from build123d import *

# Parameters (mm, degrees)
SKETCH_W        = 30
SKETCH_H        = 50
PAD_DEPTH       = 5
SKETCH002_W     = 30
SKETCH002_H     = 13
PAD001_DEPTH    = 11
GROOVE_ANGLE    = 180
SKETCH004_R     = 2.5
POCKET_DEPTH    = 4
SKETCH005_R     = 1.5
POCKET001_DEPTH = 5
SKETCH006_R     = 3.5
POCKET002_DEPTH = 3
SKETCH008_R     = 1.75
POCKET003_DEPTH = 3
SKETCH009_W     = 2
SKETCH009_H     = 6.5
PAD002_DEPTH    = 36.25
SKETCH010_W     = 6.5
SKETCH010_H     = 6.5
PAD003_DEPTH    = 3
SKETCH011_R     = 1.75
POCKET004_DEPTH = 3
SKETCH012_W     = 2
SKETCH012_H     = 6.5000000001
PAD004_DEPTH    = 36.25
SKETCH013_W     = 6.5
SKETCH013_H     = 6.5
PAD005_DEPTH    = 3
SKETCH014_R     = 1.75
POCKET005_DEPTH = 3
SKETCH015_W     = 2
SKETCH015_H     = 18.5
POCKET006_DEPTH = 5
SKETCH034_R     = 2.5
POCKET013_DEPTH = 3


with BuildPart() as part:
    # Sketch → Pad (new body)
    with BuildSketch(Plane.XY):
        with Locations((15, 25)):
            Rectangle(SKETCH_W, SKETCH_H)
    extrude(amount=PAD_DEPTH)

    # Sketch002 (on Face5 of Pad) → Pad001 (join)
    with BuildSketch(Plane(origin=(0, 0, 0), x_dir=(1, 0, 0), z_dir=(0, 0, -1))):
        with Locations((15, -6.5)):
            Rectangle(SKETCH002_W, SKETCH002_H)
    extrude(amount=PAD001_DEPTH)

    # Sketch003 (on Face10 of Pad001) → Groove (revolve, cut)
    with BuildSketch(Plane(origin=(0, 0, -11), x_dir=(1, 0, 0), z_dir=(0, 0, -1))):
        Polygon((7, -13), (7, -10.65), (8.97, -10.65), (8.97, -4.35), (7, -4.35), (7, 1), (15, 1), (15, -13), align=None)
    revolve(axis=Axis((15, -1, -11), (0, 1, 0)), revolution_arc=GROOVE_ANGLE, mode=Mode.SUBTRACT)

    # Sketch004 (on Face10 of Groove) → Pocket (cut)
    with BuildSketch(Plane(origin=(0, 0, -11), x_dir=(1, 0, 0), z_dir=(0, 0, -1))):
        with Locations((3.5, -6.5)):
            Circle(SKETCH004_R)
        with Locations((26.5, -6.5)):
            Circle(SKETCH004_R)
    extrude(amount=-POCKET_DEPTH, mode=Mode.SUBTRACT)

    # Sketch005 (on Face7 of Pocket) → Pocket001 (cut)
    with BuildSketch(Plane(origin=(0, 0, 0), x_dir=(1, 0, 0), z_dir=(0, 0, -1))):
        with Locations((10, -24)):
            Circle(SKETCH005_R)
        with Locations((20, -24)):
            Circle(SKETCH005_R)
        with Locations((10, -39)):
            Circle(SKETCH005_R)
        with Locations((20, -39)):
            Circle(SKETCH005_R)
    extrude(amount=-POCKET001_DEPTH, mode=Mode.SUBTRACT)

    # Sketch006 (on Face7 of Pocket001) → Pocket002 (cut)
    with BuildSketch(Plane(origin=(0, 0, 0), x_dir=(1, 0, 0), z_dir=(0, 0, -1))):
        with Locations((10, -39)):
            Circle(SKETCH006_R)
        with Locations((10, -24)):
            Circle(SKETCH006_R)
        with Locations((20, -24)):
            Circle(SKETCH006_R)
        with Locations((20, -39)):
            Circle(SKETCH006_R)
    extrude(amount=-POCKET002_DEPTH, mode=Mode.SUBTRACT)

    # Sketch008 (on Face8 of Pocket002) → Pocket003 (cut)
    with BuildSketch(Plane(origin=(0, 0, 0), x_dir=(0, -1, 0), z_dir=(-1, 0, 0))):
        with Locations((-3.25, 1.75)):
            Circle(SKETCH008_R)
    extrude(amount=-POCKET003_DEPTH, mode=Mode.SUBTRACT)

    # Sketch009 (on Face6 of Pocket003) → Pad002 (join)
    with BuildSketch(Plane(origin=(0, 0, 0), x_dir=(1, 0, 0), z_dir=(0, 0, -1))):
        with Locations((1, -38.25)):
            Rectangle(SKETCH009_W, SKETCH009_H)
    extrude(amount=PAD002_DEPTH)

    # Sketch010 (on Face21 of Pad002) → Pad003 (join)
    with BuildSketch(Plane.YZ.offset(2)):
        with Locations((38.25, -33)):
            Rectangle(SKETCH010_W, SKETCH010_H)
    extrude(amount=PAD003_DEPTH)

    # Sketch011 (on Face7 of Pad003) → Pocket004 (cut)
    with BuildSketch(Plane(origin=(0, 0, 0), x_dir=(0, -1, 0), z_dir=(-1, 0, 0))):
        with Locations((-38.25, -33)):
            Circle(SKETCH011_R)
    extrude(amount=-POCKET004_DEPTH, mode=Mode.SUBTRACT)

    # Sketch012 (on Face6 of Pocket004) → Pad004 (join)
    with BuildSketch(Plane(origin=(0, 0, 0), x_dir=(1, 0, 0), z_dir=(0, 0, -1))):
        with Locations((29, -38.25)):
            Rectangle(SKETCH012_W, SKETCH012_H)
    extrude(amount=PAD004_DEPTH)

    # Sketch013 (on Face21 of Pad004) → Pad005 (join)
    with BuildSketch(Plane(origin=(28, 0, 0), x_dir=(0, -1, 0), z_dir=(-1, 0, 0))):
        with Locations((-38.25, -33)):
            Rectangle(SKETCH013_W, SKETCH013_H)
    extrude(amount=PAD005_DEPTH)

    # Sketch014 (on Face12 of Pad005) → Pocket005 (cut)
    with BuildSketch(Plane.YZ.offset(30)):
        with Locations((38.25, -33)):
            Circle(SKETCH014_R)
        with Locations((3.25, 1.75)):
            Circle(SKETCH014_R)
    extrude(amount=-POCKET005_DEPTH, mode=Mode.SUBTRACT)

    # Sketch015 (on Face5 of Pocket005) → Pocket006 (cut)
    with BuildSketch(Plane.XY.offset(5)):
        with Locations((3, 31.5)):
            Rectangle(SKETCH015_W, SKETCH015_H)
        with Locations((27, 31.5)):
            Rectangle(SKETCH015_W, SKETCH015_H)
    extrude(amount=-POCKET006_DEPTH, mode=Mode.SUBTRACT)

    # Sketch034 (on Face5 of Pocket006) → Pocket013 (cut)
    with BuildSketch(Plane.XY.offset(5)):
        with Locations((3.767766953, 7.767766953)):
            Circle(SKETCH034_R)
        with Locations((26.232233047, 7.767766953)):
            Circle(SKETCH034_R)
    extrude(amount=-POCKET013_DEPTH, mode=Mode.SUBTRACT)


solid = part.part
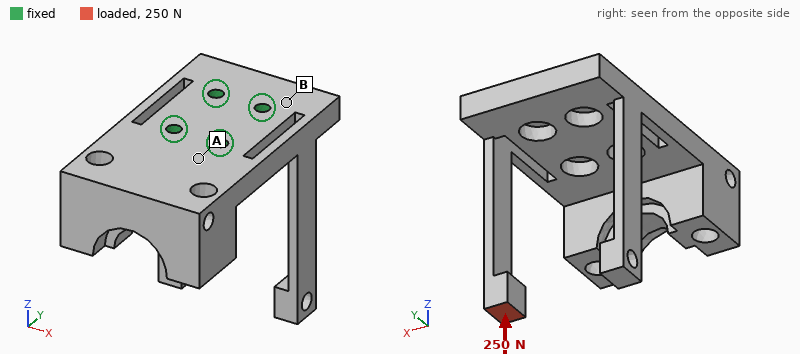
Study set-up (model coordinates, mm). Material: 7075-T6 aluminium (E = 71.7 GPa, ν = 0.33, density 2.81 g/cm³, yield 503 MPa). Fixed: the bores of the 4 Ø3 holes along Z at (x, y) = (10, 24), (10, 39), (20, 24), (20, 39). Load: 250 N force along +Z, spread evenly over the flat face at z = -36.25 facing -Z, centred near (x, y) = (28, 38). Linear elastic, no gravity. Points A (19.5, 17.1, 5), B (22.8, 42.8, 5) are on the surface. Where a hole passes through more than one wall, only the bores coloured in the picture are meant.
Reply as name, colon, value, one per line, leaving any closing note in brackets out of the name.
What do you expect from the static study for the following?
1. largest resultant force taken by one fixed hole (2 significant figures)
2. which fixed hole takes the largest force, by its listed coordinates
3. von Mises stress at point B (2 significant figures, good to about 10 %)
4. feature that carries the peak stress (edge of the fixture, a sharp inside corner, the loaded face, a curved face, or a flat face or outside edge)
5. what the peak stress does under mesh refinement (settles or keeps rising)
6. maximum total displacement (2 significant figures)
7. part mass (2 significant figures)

largest resultant force taken by one fixed hole: 310 N
which fixed hole takes the largest force, by its listed coordinates: (20, 39)
von Mises stress at point B: 21 MPa
feature that carries the peak stress: a sharp inside corner
what the peak stress does under mesh refinement: keeps rising
maximum total displacement: 0.84 mm
part mass: 30 g
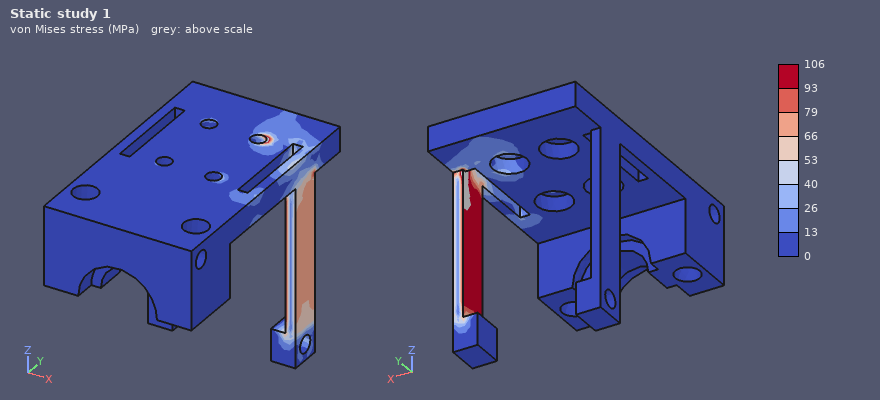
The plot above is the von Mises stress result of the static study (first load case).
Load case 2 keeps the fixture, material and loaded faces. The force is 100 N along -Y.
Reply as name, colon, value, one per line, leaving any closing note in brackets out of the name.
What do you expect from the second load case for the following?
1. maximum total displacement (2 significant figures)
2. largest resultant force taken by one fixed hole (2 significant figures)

maximum total displacement: 0.83 mm
largest resultant force taken by one fixed hole: 310 N
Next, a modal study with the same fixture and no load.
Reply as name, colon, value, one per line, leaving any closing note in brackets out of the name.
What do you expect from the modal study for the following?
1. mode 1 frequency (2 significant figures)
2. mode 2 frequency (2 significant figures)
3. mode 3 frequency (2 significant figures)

mode 1 frequency: 840 Hz
mode 2 frequency: 840 Hz
mode 3 frequency: 2300 Hz
